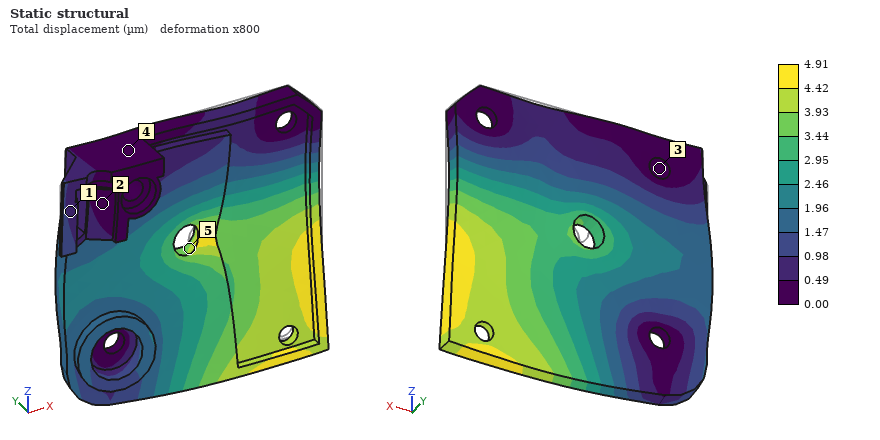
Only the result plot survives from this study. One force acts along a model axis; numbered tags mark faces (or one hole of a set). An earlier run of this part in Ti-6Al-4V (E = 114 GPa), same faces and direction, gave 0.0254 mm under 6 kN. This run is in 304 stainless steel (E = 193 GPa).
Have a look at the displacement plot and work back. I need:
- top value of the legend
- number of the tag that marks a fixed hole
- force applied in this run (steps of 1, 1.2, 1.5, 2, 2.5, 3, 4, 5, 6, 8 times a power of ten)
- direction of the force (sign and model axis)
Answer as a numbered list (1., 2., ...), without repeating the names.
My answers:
1. 4.91 µm
2. 3
3. 2 kN
4. -X
